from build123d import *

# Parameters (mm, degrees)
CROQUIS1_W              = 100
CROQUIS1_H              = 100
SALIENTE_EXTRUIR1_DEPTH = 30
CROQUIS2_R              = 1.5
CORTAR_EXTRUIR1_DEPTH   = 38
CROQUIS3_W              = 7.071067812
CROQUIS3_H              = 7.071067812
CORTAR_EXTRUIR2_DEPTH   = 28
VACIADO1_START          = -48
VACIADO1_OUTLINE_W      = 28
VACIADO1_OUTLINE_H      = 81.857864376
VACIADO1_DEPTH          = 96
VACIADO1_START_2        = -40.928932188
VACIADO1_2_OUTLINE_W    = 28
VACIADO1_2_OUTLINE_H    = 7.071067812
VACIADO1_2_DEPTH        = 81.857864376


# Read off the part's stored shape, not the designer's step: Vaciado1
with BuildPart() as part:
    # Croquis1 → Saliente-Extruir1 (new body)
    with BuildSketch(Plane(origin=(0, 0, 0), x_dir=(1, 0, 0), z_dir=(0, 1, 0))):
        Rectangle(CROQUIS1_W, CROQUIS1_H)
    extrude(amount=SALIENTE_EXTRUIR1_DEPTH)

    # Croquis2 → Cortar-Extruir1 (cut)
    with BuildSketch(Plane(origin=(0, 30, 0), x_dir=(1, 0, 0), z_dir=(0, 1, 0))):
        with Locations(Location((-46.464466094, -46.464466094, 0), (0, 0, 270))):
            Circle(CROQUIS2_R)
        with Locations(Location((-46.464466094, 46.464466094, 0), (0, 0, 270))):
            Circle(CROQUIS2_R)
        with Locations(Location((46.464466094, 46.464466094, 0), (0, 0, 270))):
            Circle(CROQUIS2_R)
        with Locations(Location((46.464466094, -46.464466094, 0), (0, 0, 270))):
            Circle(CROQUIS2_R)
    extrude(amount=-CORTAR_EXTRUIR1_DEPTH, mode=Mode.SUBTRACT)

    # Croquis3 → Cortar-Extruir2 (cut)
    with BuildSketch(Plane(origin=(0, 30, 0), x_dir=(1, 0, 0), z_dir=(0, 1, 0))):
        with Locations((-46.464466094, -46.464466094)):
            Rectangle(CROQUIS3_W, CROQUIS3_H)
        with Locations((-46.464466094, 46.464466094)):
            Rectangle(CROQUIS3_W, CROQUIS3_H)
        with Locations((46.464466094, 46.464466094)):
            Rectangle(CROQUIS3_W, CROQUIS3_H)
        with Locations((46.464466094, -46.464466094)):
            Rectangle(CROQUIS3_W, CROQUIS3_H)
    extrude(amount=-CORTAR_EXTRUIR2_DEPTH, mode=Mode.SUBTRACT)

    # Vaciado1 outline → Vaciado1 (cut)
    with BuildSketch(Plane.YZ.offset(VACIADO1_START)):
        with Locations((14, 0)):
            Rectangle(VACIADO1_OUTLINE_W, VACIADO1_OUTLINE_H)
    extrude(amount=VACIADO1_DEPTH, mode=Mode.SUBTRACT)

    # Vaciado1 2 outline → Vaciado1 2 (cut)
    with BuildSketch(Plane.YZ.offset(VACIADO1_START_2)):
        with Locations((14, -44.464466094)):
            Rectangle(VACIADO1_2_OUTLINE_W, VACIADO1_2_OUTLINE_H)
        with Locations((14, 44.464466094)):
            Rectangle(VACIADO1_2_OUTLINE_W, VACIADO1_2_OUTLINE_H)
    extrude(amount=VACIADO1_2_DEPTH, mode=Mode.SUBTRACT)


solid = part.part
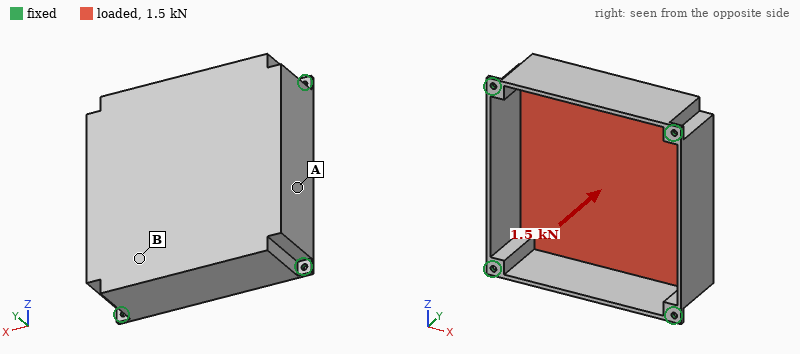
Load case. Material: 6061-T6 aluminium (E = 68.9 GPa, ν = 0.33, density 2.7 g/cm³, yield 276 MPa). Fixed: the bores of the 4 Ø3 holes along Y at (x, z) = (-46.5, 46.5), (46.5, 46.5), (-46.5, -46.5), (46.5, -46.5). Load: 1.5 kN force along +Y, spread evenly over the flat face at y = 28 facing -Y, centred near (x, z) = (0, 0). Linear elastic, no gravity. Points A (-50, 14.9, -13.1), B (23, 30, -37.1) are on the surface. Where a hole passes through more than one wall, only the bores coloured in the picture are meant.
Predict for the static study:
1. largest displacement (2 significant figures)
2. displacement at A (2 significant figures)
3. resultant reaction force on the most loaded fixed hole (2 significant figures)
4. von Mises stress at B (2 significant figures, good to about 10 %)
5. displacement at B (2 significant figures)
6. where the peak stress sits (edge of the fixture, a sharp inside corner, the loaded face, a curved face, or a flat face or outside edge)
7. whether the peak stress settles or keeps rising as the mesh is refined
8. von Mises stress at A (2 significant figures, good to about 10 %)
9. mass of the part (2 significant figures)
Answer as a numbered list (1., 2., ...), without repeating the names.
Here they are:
1. 0.62 mm
2. 0.11 mm
3. 410 N
4. 40 MPa
5. 0.14 mm
6. edge of the fixture
7. keeps rising
8. 24 MPa
9. 110 g
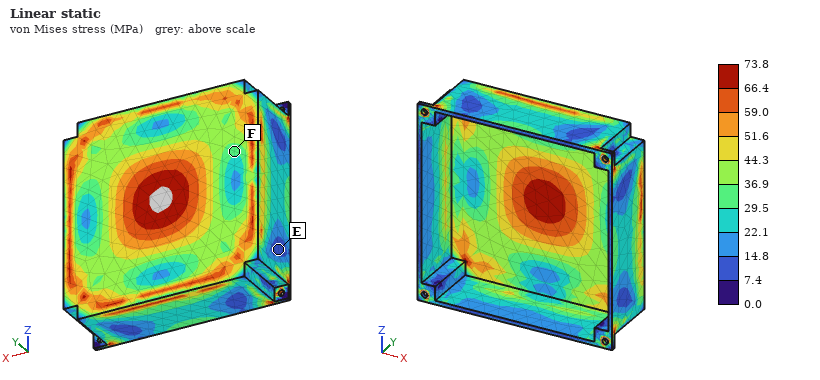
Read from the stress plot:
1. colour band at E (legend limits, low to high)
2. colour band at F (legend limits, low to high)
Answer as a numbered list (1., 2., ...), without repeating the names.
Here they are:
1. 7.4 to 14.8 MPa
2. 29.5 to 36.9 MPa
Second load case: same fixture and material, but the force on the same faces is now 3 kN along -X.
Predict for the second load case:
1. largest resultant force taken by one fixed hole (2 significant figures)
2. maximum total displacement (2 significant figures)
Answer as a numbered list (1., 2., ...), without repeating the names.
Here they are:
1. 870 N
2. 41 µm
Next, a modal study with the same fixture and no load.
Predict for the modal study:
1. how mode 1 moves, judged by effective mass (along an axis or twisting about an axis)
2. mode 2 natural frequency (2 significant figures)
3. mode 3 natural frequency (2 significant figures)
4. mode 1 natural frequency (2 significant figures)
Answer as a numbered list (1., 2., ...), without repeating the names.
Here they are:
1. along Y
2. 2300 Hz
3. 2300 Hz
4. 1400 Hz
